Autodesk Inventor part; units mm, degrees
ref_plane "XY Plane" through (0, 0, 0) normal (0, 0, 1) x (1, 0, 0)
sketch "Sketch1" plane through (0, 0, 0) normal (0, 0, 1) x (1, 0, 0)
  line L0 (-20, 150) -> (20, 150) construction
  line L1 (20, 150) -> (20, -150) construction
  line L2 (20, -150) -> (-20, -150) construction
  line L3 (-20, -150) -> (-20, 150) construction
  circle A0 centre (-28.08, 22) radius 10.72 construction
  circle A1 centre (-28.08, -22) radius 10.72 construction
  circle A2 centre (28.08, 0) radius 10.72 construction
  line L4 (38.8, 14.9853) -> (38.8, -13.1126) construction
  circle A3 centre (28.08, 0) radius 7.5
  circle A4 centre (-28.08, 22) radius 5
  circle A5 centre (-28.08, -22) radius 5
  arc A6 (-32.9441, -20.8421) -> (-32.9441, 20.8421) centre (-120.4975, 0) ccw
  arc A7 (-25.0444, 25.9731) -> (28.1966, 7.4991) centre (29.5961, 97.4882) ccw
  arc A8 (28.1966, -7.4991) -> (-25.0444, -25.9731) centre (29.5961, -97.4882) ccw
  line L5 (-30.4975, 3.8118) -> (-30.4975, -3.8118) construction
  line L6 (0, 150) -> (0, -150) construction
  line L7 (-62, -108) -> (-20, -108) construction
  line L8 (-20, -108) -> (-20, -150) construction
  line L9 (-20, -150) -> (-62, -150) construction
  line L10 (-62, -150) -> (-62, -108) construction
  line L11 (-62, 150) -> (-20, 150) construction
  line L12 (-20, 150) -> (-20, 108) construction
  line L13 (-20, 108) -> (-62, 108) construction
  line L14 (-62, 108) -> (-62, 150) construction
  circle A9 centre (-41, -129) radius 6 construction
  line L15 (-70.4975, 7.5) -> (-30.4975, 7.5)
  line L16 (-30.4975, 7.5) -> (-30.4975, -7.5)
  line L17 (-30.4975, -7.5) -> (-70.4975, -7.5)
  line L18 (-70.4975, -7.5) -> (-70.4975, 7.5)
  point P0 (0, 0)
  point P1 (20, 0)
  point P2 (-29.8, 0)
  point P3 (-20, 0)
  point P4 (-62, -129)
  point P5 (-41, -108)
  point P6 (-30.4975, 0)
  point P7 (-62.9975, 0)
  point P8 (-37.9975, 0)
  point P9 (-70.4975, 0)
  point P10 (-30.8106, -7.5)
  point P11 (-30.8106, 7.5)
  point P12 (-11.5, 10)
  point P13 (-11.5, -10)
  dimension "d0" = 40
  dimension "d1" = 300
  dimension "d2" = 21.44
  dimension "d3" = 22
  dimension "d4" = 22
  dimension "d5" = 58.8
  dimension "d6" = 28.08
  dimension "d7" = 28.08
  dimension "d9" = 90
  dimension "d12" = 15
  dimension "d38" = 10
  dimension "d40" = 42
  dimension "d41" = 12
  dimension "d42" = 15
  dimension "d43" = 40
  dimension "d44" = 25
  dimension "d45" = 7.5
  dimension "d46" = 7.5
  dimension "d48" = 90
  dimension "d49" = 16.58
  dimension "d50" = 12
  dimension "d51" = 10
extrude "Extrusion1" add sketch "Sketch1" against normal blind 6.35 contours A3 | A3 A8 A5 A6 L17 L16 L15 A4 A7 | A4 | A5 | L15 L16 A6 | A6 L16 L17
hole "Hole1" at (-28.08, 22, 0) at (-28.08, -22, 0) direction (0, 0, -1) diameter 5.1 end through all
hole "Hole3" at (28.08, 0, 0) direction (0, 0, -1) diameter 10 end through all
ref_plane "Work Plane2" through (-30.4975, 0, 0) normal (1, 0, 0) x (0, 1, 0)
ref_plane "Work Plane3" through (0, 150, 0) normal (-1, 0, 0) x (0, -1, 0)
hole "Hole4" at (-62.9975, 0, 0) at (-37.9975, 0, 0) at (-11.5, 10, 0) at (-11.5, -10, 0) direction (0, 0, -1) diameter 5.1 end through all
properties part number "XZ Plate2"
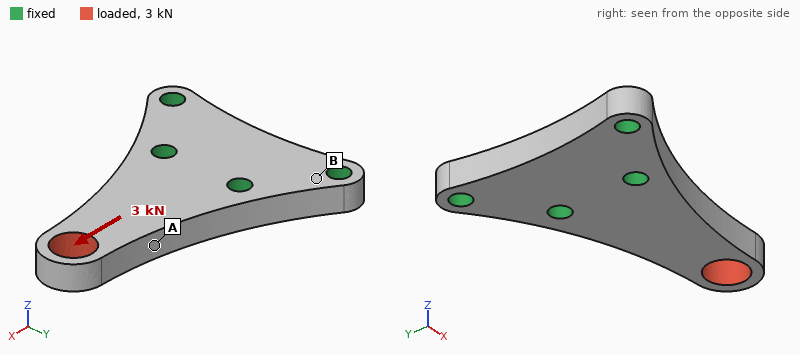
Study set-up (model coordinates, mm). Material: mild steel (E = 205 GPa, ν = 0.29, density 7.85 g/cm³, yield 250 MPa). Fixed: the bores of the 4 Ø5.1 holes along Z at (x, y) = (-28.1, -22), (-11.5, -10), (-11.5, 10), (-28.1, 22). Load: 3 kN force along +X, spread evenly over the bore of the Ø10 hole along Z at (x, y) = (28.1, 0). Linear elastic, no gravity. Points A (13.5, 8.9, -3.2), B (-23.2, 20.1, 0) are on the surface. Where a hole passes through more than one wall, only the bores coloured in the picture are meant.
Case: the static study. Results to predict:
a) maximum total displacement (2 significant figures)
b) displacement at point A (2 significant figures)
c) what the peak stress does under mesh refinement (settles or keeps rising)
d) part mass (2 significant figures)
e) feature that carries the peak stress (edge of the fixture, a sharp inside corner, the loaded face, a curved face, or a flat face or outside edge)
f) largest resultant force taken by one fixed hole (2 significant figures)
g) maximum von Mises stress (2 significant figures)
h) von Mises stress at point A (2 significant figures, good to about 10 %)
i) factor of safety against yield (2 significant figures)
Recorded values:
11 µm
2.5 µm
settles
85 g
the loaded face
1.5 kN
130 MPa
32 MPa
1.9
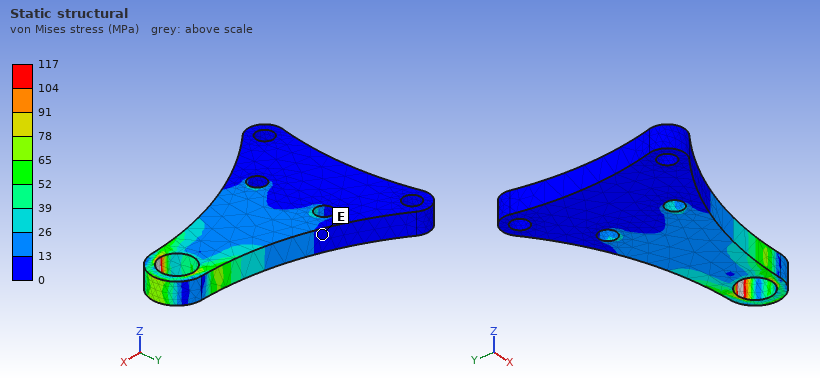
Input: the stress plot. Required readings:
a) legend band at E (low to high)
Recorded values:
0 to 13 MPa
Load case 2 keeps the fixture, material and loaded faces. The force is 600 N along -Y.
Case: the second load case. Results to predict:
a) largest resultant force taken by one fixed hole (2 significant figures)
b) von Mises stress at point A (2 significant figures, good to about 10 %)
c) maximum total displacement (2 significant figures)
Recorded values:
1.0 kN
29 MPa
18 µm
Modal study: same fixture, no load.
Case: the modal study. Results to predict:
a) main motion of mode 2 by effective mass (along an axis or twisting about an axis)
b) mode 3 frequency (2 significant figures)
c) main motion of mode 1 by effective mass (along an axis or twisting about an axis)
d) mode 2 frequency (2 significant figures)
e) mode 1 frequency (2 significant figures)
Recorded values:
along Y
16 kHz
along Z
12 kHz
3900 Hz
